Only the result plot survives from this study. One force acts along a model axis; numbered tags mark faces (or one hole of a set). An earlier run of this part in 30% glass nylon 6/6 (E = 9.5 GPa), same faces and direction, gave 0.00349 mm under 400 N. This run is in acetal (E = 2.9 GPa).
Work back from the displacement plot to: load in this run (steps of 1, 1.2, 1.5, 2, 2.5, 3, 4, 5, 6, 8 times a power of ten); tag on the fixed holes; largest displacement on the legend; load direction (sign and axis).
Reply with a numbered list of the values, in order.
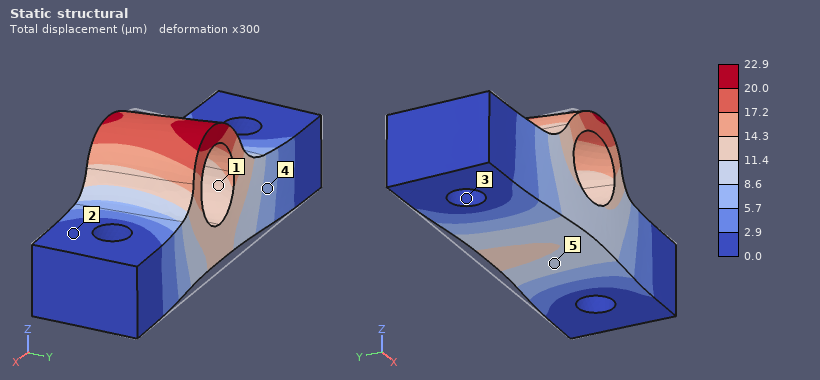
1. 800 N
2. 3
3. 22.9 µm
4. -Y
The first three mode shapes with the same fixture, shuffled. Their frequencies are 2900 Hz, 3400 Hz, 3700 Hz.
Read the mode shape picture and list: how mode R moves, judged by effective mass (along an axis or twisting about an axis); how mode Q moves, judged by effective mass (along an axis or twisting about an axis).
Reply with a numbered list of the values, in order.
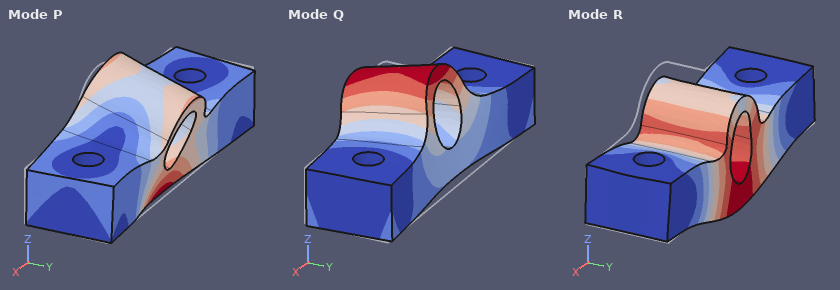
1. along Z
2. along Y
